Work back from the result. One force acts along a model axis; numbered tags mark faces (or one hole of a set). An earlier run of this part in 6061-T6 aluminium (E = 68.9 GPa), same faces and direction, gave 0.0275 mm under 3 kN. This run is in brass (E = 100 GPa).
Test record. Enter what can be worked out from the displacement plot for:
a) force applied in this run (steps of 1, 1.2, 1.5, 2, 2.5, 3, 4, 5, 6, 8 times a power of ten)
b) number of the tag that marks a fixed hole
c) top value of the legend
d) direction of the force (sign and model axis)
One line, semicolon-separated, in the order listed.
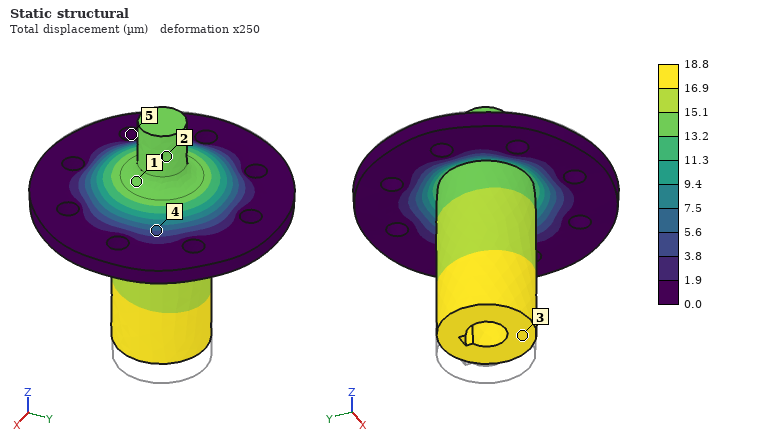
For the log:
3 kN; 5; 18.8 µm; +Z
